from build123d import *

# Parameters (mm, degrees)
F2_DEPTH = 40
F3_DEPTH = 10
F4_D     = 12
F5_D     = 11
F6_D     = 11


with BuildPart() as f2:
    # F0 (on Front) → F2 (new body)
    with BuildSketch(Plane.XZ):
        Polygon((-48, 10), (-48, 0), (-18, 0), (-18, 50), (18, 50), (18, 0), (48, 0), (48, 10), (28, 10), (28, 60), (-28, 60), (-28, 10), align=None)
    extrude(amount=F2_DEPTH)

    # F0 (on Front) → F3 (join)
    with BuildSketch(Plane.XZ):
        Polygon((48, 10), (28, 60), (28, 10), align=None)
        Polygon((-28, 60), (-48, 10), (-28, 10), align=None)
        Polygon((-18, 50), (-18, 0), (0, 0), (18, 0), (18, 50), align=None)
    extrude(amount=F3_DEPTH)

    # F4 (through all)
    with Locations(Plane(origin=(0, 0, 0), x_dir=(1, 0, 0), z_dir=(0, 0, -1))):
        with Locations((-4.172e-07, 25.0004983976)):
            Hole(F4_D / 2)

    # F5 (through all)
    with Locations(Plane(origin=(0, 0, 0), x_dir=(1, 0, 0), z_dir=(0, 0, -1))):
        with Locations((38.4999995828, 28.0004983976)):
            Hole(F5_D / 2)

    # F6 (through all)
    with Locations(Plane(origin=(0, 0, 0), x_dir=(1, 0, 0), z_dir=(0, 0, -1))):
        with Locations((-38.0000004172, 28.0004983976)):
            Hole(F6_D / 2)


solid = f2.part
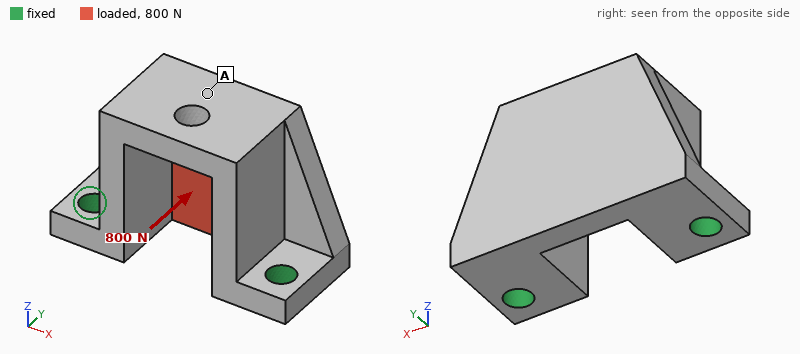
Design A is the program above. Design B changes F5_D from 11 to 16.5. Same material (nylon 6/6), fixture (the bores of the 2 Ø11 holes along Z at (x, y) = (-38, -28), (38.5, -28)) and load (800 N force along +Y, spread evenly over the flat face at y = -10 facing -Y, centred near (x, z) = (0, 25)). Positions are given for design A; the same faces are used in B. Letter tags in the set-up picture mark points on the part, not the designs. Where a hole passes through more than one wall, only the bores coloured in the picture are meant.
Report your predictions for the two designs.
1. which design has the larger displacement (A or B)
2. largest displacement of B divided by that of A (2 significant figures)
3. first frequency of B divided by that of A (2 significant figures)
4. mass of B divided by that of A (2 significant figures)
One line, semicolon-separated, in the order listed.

A; 0.81; 1.1; 0.99
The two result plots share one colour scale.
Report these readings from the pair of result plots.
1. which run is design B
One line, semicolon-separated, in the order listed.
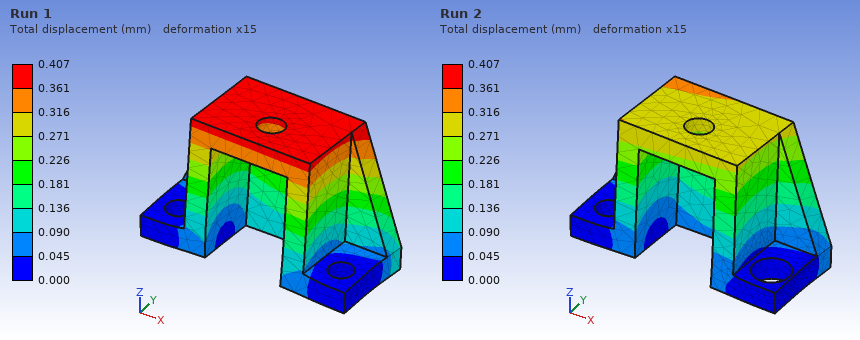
Run 2
